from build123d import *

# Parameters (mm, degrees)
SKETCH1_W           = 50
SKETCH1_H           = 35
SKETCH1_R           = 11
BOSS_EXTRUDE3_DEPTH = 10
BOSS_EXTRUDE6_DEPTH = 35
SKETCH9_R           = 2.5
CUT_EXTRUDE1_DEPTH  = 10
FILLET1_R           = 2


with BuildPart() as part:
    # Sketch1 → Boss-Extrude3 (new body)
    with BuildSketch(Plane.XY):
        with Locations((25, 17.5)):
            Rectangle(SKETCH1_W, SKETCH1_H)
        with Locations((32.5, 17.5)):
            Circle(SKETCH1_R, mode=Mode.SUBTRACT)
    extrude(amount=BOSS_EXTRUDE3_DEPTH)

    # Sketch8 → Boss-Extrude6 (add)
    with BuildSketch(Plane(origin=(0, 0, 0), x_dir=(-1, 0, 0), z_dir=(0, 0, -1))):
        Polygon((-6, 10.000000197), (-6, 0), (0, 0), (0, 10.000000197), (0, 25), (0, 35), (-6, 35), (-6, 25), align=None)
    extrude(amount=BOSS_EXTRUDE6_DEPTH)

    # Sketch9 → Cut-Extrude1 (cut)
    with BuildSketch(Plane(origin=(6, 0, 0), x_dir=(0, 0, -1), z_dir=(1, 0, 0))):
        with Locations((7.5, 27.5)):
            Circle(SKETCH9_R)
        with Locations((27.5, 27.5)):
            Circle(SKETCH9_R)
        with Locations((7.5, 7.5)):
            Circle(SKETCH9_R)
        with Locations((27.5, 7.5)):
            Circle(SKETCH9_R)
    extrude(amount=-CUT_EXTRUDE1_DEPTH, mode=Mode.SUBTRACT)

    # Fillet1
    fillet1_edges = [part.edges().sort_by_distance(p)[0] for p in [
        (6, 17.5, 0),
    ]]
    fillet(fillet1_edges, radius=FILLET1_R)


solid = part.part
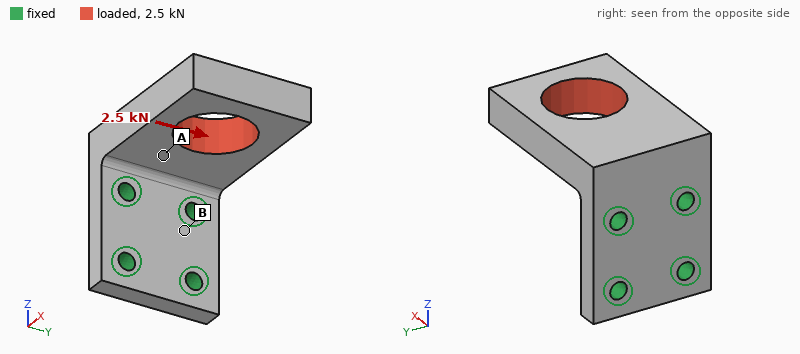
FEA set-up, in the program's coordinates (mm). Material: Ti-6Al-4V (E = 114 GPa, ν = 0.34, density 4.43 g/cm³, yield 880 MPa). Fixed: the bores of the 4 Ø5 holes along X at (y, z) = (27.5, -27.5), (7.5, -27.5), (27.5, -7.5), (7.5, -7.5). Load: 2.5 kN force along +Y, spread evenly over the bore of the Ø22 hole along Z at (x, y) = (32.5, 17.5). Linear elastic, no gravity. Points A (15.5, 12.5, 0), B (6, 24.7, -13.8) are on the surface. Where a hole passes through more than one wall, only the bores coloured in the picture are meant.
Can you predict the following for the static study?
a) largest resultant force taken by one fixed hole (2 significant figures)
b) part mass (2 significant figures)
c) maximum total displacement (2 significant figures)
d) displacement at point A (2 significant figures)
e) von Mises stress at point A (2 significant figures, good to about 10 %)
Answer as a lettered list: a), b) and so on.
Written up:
a) 3.5 kN
b) 91 g
c) 0.12 mm
d) 0.028 mm
e) 47 MPa
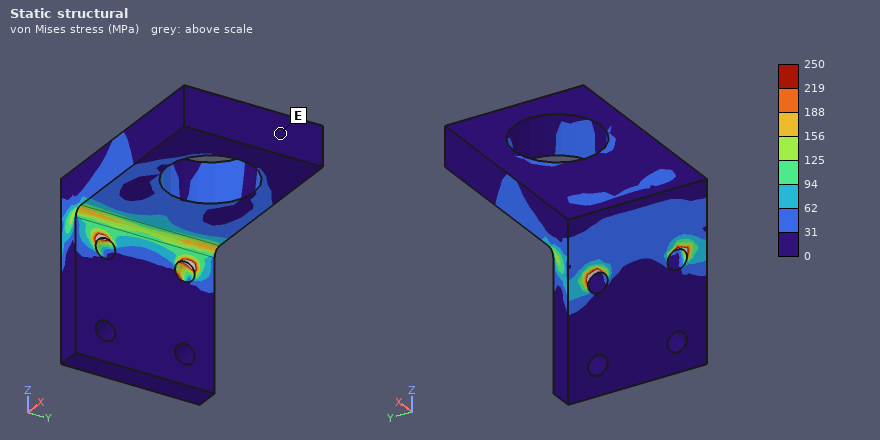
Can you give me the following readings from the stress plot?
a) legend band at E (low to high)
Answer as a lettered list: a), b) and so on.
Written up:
a) 0 to 31 MPa
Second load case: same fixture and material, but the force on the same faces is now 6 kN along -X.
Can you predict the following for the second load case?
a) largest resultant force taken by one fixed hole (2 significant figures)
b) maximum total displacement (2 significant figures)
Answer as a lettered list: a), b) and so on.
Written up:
a) 3.3 kN
b) 0.27 mm
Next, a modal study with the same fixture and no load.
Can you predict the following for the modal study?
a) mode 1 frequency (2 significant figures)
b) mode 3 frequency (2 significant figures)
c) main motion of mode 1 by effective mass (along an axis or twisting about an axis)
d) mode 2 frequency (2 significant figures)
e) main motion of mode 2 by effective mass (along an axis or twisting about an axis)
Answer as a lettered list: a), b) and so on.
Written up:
a) 2000 Hz
b) 7400 Hz
c) along Z
d) 4200 Hz
e) along Y
